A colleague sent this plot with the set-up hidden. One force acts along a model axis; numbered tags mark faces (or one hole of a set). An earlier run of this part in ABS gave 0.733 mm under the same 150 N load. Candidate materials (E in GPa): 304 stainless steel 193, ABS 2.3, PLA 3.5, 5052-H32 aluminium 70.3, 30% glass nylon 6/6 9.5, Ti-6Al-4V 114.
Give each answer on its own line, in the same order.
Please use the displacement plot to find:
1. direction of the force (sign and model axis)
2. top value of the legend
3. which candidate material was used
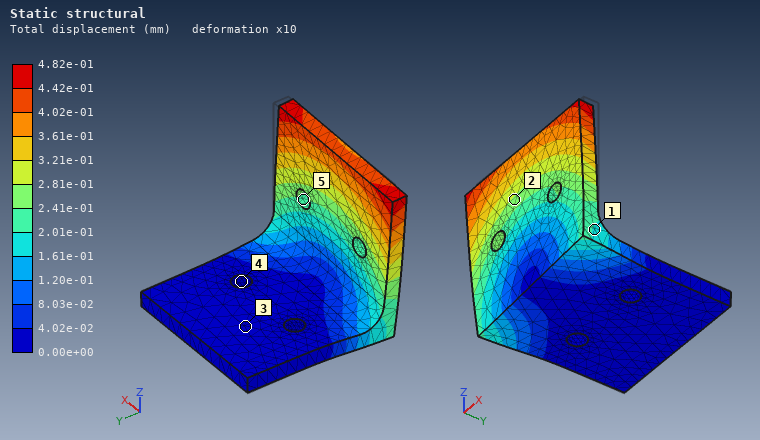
-X
4.82e-01 mm
PLA
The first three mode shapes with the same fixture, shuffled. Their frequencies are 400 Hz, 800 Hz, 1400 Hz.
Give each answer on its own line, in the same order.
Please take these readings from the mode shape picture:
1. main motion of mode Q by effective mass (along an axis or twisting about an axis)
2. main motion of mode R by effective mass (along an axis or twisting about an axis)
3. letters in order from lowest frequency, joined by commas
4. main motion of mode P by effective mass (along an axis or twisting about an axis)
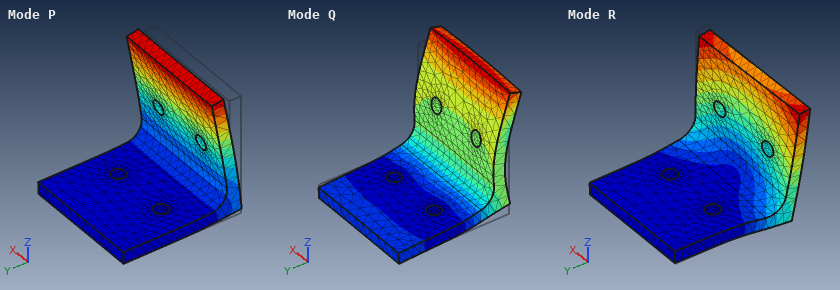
along Z
along X
P, R, Q
along Y
